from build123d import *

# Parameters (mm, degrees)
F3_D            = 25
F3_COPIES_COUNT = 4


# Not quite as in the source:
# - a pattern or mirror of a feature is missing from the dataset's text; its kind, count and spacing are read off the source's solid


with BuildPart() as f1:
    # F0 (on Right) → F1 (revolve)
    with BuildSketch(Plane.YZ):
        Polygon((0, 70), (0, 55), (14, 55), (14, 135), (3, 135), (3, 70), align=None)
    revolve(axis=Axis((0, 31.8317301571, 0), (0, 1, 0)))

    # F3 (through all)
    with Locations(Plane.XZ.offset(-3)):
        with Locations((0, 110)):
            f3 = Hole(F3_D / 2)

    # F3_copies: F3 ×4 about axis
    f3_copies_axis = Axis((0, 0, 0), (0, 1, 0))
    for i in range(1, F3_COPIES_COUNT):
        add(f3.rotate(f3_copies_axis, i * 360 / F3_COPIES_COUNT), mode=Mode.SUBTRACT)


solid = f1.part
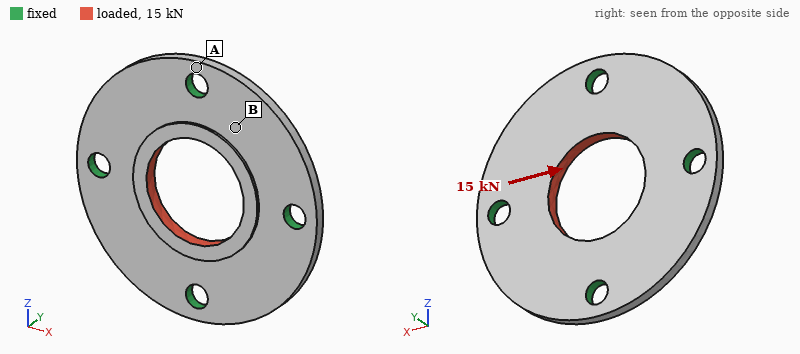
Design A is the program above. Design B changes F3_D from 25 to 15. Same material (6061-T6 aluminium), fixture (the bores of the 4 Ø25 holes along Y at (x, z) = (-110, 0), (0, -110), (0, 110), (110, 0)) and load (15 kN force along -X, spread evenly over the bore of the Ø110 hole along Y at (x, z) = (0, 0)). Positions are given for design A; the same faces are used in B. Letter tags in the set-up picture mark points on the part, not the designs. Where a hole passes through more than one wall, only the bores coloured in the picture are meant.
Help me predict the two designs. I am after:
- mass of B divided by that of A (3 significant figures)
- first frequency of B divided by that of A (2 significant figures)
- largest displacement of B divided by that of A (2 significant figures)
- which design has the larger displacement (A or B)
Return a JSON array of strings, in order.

["1.03", "0.83", "1.1", "B"]
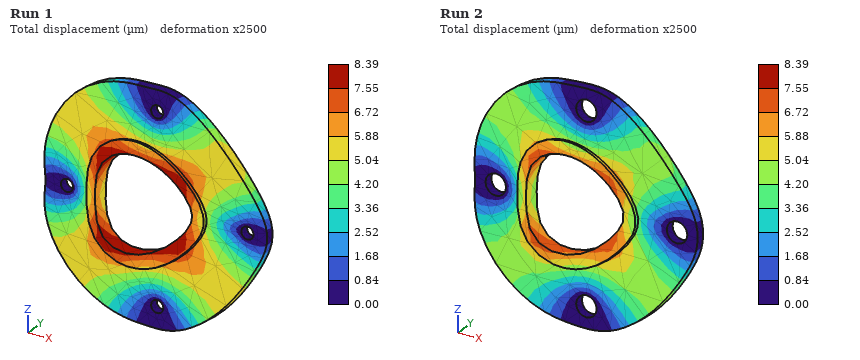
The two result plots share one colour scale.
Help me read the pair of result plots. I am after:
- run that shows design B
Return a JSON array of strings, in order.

["Run 1"]
